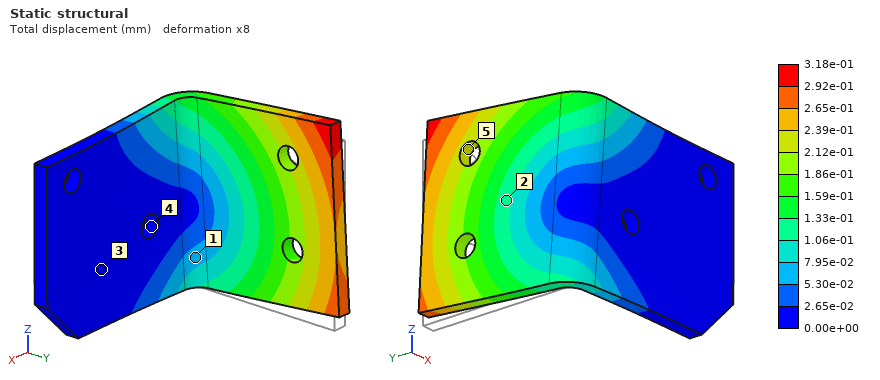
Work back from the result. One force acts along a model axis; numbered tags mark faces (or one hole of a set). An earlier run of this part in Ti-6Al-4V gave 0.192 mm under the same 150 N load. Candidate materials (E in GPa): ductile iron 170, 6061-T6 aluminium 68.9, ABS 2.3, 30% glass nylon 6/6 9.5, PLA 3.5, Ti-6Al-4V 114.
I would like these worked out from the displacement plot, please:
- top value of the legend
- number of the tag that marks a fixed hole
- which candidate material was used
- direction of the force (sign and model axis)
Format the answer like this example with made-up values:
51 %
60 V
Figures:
3.18e-01 mm
4
6061-T6 aluminium
+Z
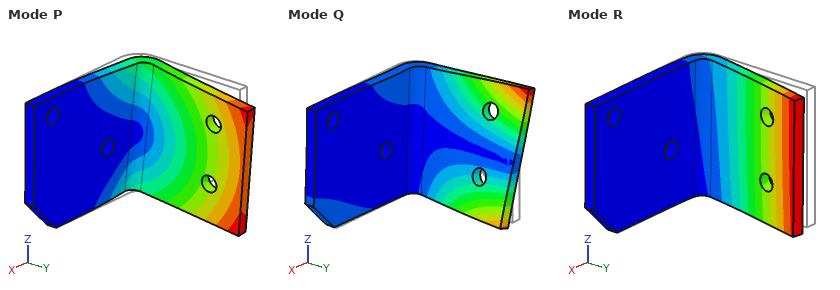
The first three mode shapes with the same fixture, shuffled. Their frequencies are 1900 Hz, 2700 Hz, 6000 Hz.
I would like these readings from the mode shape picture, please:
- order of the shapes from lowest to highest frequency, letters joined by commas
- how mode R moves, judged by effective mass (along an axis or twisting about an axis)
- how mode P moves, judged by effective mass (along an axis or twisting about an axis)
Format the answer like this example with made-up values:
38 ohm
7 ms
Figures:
R, P, Q
along X
along Z
